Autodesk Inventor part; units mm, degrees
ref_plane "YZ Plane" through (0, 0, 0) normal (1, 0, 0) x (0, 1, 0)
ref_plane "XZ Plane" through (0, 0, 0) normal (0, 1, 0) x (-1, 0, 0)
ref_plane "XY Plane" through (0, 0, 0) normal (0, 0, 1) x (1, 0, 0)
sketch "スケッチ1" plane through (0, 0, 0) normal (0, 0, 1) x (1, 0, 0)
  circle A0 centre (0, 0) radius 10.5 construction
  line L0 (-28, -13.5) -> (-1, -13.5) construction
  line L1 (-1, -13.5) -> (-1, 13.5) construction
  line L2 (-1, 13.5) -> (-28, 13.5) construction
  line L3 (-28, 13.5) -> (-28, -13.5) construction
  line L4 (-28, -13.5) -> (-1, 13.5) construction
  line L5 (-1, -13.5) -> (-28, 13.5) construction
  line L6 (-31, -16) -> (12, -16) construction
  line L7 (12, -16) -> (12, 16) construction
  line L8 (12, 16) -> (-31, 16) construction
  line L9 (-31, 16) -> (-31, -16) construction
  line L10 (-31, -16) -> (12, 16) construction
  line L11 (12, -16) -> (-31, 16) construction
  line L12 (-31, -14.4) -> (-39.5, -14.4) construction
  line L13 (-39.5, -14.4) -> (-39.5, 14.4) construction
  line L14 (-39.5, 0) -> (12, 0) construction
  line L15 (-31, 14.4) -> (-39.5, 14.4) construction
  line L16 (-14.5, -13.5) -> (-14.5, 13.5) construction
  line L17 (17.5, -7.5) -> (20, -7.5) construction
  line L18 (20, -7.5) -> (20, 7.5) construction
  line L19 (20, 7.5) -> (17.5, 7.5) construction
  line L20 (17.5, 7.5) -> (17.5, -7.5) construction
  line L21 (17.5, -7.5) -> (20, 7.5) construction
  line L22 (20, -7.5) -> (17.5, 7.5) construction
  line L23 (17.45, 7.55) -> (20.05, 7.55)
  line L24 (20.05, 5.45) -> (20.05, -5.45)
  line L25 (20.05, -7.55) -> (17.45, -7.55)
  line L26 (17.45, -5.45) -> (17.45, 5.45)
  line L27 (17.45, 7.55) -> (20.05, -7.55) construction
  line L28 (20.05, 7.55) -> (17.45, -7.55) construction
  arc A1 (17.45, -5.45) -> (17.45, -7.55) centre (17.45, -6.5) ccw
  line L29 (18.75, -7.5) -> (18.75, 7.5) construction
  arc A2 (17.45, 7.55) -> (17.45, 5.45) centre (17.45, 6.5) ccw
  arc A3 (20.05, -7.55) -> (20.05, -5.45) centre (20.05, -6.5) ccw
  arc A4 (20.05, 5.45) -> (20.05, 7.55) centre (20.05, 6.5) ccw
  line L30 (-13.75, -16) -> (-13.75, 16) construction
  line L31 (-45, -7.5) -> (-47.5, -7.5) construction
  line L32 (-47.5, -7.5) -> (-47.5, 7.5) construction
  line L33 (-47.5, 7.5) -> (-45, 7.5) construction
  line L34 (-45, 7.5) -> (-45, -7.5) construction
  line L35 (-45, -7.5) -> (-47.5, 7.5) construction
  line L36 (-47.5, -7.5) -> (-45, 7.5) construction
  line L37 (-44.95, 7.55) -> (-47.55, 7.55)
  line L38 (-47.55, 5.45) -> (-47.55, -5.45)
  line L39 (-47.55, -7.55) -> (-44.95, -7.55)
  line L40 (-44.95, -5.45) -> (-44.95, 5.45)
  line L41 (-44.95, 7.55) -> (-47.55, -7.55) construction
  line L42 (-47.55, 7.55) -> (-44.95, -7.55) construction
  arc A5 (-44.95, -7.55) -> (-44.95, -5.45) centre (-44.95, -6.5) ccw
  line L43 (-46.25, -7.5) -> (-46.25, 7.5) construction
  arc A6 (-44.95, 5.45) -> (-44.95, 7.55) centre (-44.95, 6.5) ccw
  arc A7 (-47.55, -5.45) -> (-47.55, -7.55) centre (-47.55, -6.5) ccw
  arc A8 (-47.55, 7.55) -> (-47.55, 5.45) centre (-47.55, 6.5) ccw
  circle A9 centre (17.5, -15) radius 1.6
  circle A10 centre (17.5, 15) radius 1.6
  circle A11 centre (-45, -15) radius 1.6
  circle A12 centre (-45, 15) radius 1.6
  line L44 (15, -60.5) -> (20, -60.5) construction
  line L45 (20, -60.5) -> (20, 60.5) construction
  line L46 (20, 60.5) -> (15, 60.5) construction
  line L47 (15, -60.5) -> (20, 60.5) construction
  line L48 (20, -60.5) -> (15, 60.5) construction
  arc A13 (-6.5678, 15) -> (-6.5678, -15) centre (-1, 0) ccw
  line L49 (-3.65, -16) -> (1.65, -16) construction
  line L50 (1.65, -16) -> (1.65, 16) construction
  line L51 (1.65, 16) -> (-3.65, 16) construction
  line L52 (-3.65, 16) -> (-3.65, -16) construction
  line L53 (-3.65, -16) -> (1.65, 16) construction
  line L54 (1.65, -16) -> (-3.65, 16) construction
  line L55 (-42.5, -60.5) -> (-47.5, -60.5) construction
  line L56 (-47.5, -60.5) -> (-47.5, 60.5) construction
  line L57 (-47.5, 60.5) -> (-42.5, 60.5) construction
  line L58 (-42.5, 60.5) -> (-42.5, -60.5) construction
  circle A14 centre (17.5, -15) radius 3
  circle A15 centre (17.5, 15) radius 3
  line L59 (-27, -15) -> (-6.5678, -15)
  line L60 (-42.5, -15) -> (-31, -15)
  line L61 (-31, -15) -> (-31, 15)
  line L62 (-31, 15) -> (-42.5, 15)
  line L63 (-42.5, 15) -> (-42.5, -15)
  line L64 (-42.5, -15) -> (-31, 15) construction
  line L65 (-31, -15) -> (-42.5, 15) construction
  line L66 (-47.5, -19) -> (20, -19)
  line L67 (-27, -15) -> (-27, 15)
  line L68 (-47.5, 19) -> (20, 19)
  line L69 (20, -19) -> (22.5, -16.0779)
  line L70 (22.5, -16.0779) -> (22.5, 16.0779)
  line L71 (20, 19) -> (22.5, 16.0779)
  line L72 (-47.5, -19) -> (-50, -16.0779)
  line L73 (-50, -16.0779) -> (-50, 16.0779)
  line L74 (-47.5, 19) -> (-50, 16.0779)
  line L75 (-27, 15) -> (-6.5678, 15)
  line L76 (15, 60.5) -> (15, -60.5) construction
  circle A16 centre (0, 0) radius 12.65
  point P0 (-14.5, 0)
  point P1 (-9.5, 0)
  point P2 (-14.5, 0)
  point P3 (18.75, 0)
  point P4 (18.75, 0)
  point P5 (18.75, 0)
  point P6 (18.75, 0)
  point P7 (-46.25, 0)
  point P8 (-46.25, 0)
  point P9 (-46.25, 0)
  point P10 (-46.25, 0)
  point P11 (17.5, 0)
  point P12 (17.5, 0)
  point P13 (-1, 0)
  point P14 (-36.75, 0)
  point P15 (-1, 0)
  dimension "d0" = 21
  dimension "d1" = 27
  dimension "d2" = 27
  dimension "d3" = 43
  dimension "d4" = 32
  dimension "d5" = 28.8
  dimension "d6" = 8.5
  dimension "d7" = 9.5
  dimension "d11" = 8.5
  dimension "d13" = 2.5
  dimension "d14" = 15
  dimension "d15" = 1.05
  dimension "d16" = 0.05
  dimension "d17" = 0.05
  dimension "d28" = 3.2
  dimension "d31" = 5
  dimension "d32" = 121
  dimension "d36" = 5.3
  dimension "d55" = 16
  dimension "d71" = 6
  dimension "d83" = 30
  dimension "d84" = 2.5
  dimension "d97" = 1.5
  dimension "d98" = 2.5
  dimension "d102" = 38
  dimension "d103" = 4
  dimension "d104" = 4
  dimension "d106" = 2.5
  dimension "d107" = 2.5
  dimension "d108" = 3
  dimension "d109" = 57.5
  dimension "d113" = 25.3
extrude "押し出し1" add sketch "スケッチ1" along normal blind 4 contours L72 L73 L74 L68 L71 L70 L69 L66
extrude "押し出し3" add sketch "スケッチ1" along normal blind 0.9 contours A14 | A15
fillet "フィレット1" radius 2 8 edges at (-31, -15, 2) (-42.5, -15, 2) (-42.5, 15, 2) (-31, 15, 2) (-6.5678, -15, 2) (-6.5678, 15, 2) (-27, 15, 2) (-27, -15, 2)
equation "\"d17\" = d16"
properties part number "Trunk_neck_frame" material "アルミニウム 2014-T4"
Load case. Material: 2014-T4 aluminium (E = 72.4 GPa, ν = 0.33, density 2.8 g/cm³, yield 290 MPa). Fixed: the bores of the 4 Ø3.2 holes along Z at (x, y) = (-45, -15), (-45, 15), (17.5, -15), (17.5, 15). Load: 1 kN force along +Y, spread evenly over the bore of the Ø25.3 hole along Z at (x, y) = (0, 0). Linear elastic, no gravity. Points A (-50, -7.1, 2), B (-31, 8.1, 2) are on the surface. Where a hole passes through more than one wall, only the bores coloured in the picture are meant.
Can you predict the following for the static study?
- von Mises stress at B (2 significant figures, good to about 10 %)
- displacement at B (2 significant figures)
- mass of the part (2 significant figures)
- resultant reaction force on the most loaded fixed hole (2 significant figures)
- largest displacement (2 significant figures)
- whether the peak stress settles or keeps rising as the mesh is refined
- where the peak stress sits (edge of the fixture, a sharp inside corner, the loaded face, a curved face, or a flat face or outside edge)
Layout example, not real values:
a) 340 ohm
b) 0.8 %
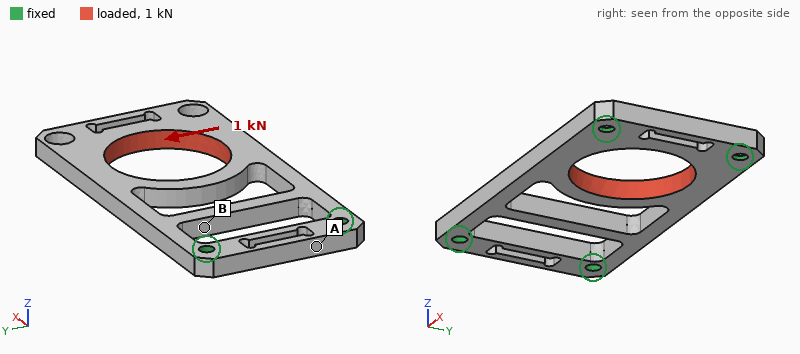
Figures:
a) 32 MPa
b) 26 µm
c) 15 g
d) 470 N
e) 55 µm
f) keeps rising
g) edge of the fixture
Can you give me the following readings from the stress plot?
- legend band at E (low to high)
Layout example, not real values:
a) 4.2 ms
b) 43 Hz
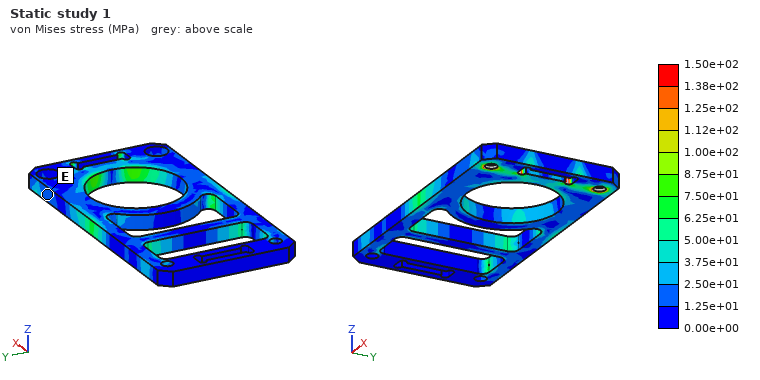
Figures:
a) 1.25e+01 to 2.50e+01 MPa
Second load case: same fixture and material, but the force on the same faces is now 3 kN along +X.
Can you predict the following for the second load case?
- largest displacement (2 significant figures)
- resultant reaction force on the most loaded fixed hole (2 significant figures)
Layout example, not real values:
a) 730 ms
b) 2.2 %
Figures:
a) 68 µm
b) 1.0 kN
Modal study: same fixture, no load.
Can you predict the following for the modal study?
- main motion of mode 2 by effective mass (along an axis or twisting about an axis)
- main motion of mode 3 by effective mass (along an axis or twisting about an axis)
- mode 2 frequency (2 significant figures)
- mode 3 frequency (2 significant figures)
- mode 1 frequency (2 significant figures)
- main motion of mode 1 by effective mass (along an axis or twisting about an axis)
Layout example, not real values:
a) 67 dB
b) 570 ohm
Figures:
a) twisting about X
b) along Y
c) 5400 Hz
d) 7400 Hz
e) 3500 Hz
f) along Z
